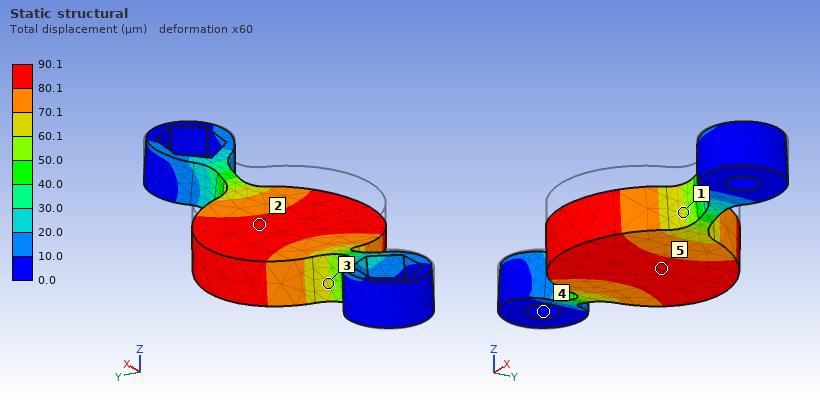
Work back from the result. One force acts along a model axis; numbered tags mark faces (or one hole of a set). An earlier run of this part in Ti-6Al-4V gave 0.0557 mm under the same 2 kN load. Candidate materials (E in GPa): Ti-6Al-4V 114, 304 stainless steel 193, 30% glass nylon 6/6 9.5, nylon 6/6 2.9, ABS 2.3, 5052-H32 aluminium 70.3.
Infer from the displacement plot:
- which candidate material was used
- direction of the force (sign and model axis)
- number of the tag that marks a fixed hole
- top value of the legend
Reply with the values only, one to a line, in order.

5052-H32 aluminium
-Z
4
90.1 µm
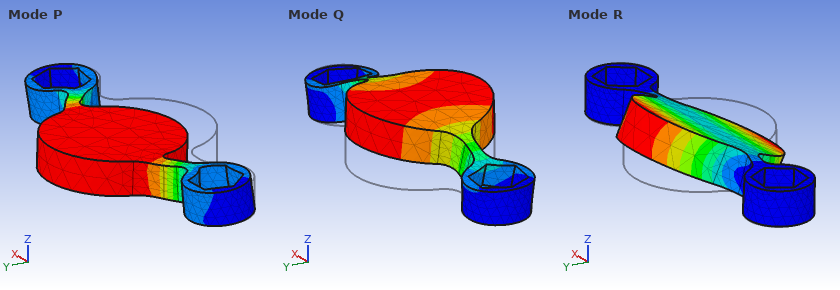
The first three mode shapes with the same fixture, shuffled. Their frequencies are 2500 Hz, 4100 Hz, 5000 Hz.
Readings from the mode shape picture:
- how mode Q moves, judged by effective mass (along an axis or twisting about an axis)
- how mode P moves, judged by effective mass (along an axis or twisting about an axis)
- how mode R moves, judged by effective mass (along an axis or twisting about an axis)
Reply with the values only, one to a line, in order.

along Z
along Y
twisting about X
